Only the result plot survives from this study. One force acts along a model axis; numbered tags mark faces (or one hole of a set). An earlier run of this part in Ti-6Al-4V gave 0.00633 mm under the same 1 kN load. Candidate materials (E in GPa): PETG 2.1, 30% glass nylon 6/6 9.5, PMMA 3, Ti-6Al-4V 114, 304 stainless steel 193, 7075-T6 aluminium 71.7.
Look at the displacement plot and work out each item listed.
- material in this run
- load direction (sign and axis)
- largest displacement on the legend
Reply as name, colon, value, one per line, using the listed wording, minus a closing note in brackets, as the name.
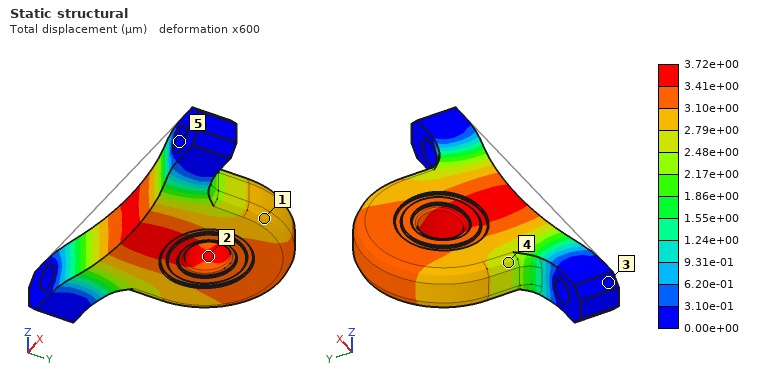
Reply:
material in this run: 304 stainless steel
load direction: +Y
largest displacement on the legend: 3.72e+00 µm
